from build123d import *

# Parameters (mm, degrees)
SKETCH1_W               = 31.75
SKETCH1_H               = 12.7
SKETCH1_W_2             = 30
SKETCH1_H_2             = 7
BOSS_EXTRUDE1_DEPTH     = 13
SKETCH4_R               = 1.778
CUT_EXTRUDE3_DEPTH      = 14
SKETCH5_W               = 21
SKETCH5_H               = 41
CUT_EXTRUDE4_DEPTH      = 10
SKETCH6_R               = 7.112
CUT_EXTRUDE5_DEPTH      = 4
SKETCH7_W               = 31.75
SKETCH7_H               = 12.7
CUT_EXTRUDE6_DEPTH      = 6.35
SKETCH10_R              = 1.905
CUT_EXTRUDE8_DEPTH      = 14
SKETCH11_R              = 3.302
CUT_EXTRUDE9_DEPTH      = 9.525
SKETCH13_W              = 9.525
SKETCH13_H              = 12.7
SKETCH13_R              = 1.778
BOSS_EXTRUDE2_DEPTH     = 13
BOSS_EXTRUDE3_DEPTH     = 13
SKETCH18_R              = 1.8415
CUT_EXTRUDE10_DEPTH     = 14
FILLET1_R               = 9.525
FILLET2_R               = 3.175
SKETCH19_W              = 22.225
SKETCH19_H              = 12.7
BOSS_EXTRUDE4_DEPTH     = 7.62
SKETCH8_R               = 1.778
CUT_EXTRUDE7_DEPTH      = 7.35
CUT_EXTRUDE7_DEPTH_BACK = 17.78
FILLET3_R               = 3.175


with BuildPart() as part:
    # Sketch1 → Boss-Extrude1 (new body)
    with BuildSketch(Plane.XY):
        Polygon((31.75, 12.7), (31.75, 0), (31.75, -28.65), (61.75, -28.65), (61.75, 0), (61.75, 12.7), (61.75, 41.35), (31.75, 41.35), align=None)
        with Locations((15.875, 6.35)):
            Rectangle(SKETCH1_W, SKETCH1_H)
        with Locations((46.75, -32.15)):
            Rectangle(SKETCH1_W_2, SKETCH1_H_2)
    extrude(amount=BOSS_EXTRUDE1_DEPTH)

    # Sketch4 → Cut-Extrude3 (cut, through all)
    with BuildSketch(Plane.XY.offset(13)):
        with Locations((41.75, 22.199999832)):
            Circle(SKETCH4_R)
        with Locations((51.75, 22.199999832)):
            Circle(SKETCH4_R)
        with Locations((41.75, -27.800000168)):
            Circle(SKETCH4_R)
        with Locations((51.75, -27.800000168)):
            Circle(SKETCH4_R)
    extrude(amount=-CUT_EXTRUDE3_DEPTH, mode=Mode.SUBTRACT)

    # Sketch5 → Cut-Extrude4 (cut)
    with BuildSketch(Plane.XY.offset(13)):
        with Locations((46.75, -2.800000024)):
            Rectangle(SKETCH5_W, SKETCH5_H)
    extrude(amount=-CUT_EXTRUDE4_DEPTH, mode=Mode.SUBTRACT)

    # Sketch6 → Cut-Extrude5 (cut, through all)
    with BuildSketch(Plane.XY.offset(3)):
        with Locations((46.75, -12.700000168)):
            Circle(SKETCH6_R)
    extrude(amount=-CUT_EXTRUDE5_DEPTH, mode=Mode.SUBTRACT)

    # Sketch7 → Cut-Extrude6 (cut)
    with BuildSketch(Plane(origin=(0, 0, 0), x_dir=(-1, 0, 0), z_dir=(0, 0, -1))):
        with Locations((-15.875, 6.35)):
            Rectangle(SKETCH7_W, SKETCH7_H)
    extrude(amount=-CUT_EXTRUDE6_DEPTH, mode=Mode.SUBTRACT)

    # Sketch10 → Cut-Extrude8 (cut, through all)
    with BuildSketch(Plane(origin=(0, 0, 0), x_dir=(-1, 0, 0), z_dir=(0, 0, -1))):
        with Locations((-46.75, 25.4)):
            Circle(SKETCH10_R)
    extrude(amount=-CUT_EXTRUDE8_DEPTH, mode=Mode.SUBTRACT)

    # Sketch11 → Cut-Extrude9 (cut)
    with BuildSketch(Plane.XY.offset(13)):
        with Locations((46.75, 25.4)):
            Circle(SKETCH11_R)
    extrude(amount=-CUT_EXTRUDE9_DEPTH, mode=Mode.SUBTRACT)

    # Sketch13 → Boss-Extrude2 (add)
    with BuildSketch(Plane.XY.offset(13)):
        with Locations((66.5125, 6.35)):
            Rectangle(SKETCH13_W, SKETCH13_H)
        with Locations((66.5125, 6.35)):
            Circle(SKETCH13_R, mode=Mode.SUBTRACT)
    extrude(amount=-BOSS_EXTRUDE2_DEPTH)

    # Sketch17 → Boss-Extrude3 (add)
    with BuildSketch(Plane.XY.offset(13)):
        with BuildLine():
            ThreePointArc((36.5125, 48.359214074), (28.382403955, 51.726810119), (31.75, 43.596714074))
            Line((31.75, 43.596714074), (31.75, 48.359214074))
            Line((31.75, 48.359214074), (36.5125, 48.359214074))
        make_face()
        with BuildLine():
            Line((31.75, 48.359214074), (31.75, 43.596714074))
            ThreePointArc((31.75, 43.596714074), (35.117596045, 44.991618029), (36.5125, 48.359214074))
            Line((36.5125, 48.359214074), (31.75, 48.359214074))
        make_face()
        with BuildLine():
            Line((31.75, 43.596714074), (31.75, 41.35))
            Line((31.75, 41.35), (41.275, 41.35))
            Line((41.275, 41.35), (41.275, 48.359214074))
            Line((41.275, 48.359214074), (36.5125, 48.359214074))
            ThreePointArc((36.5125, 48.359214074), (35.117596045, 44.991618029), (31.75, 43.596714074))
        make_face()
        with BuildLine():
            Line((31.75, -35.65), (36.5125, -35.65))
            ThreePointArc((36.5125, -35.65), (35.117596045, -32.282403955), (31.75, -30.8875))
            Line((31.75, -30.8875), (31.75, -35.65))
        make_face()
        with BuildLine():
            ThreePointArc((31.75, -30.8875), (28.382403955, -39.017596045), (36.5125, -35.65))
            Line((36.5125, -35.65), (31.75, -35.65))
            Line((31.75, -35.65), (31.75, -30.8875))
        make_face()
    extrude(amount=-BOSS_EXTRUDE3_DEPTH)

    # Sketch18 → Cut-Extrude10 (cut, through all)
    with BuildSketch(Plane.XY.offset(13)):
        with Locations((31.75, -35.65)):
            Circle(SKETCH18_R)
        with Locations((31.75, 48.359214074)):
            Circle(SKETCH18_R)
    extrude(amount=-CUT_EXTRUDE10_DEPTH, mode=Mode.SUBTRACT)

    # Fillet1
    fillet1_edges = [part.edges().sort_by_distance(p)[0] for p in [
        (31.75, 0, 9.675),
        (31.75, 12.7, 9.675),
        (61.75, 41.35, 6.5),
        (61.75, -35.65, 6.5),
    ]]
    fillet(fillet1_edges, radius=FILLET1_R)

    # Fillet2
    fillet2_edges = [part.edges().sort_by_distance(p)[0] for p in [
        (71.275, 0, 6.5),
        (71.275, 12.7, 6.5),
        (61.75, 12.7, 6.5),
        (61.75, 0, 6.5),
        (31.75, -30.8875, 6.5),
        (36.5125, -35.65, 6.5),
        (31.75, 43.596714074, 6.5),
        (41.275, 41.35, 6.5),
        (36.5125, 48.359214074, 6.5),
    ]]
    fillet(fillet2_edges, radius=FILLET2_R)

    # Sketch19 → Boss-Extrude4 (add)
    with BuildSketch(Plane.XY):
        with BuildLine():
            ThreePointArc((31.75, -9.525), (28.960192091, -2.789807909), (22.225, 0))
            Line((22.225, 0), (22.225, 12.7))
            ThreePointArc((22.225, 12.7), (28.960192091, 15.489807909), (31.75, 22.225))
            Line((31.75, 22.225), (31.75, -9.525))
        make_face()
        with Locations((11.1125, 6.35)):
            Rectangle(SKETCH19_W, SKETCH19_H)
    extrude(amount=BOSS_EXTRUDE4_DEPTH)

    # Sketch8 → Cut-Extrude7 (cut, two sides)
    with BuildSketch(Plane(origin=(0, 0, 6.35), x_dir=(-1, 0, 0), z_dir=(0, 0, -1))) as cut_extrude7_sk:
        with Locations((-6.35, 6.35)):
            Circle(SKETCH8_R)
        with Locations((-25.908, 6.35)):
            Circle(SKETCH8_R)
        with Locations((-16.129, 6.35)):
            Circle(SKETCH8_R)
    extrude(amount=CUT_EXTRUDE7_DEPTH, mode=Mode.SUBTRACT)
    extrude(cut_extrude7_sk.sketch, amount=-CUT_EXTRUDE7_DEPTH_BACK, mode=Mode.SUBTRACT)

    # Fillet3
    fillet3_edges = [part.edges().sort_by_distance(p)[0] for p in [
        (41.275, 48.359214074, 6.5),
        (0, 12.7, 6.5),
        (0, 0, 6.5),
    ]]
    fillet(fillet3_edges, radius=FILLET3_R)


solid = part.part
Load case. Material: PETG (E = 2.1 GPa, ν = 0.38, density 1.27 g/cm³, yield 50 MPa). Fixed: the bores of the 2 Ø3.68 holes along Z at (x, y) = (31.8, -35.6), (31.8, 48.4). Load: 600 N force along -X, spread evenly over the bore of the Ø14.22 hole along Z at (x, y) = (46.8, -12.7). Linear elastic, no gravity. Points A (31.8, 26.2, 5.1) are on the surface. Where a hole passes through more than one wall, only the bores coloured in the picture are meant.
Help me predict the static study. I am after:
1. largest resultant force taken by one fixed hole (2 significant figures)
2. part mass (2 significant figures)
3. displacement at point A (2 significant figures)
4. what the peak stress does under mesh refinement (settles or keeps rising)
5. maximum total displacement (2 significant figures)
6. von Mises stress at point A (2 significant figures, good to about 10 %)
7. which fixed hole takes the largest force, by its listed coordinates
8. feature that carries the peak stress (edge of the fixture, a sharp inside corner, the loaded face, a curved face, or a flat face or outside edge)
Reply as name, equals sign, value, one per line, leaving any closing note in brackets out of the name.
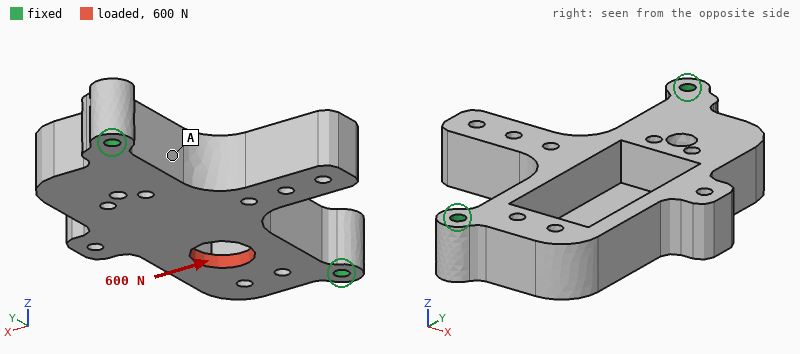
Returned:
largest resultant force taken by one fixed hole = 480 N
part mass = 36 g
displacement at point A = 0.085 mm
what the peak stress does under mesh refinement = keeps rising
maximum total displacement = 0.39 mm
von Mises stress at point A = 2.0 MPa
which fixed hole takes the largest force, by its listed coordinates = (31.8, -35.6)
feature that carries the peak stress = edge of the fixture
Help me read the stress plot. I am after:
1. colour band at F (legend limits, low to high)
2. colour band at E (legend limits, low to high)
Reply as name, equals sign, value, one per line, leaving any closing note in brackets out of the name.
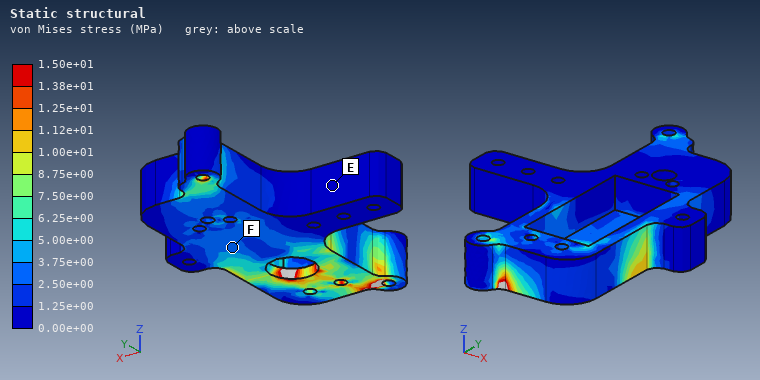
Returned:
colour band at F = 2.50e+00 to 3.75e+00 MPa
colour band at E = 0.00e+00 to 1.25e+00 MPa
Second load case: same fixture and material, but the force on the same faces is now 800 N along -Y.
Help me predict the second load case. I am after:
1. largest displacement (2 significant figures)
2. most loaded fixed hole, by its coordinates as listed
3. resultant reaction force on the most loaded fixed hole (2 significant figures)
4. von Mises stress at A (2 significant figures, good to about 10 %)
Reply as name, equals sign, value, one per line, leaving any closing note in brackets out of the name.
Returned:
largest displacement = 0.16 mm
most loaded fixed hole, by its coordinates as listed = (31.8, -35.6)
resultant reaction force on the most loaded fixed hole = 460 N
von Mises stress at A = 3.5 MPa
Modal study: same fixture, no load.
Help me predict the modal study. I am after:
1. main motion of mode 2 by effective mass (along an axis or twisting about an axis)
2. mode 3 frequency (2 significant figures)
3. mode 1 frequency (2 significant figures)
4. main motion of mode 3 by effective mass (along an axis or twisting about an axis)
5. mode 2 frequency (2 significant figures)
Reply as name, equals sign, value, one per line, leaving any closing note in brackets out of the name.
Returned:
main motion of mode 2 by effective mass = along Z
mode 3 frequency = 1700 Hz
mode 1 frequency = 700 Hz
main motion of mode 3 by effective mass = along X
mode 2 frequency = 1100 Hz
